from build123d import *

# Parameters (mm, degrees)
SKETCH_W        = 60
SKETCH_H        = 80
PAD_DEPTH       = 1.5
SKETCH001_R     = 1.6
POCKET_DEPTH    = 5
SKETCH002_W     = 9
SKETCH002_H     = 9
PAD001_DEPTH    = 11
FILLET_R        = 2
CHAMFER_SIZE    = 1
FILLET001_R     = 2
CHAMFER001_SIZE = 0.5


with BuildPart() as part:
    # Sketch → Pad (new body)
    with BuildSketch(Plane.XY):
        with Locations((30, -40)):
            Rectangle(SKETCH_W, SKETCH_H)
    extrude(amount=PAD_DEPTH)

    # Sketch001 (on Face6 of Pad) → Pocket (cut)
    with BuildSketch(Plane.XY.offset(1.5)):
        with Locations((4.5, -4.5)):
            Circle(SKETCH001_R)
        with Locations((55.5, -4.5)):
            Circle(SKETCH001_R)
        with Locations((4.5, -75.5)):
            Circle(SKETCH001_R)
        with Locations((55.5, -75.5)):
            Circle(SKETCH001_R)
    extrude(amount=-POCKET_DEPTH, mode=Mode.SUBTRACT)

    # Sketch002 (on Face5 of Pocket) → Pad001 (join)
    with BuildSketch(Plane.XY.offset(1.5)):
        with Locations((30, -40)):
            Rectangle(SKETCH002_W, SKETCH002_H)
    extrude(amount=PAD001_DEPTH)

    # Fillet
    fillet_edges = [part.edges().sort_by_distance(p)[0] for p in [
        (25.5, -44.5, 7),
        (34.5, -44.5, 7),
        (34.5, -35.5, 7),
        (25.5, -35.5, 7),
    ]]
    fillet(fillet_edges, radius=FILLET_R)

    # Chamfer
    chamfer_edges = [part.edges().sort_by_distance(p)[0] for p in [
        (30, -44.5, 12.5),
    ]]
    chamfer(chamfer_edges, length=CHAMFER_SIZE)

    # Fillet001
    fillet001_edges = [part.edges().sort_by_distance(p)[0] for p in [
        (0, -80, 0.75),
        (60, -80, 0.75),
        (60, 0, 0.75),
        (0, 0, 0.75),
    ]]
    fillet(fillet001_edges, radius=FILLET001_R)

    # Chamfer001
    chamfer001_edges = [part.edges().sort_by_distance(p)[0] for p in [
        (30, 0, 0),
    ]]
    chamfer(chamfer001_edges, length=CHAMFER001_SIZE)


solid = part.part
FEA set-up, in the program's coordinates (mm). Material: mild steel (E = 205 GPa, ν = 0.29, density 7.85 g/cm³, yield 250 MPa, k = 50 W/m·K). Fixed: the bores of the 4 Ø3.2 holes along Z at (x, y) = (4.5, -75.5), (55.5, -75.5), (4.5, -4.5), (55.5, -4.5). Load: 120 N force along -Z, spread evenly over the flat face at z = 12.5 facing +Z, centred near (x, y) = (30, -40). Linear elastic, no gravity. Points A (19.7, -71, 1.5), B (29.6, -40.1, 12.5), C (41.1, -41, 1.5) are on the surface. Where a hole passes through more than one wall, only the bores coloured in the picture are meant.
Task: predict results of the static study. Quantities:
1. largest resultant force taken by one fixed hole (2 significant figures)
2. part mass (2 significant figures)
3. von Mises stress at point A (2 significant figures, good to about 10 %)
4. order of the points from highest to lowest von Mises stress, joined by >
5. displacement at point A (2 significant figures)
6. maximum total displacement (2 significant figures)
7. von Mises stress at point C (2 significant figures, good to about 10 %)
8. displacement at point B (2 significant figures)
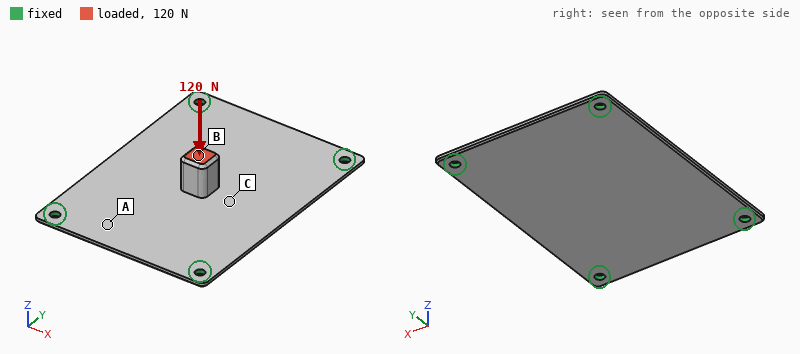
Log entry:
30 N
62 g
18 MPa
C > A > B
20 µm
98 µm
36 MPa
98 µm
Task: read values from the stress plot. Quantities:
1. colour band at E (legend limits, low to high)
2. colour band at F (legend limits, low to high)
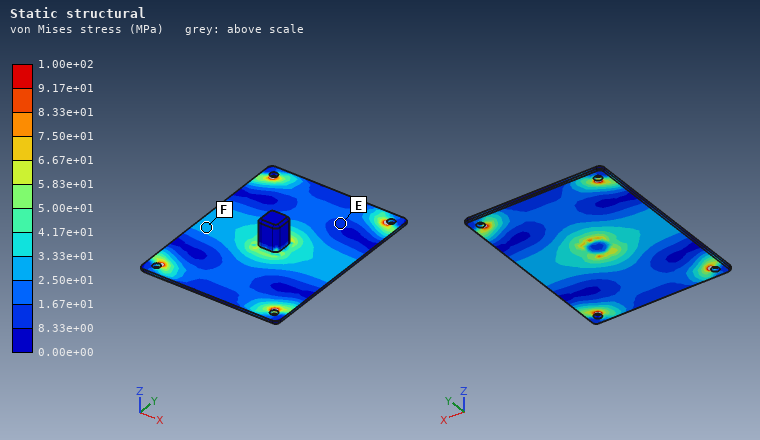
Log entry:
8.33e+00 to 1.67e+01 MPa
2.50e+01 to 3.33e+01 MPa
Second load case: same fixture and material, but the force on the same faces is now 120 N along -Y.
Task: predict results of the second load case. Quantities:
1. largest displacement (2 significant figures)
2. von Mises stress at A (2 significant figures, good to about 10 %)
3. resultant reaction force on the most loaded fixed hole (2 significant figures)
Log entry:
34 µm
5.0 MPa
35 N
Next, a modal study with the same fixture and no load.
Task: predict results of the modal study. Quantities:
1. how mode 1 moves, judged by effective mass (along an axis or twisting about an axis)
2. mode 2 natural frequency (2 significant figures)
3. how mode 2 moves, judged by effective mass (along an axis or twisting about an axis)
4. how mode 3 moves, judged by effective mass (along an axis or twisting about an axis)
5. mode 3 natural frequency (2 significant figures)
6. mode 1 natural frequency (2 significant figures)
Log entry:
along Z
2000 Hz
twisting about Y
twisting about X
2800 Hz
1100 Hz
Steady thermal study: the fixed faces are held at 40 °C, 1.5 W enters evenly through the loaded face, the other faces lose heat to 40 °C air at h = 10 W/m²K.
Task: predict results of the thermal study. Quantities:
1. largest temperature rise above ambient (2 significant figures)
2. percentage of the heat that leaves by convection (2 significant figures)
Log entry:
14 K
26 %
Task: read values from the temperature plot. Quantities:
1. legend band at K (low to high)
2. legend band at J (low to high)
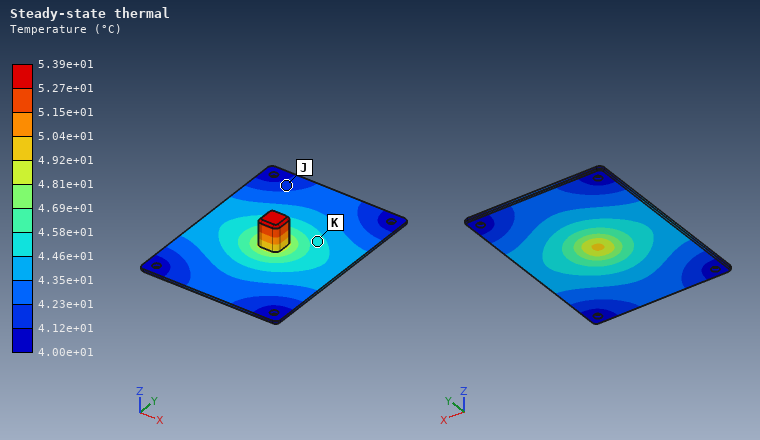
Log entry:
4.46e+01 to 4.58e+01 °C
4.12e+01 to 4.23e+01 °C
